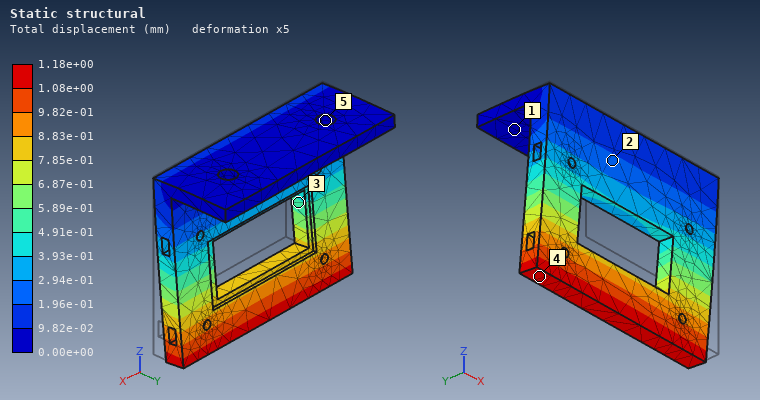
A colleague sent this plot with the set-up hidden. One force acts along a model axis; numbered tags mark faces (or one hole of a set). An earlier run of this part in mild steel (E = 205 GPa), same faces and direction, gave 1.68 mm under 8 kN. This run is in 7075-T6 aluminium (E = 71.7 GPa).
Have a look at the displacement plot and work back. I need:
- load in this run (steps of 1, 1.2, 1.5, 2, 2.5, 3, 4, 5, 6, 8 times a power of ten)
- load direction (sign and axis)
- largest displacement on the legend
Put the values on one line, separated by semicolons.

2 kN; +Y; 1.18e+00 mm
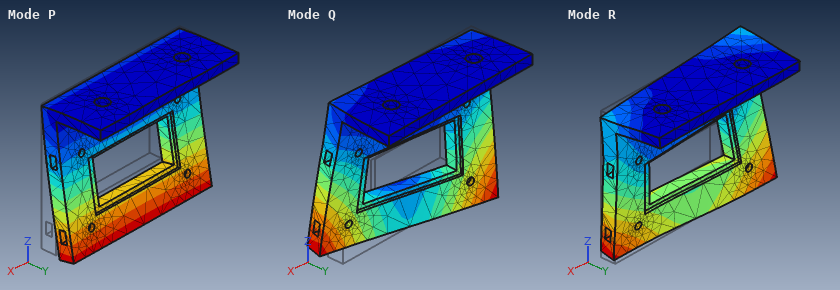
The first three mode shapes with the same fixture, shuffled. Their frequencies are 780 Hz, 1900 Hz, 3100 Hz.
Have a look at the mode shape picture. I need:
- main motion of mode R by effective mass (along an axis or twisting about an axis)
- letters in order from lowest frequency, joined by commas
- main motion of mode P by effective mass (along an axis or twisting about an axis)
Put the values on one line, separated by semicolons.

along X; P, Q, R; along Y
